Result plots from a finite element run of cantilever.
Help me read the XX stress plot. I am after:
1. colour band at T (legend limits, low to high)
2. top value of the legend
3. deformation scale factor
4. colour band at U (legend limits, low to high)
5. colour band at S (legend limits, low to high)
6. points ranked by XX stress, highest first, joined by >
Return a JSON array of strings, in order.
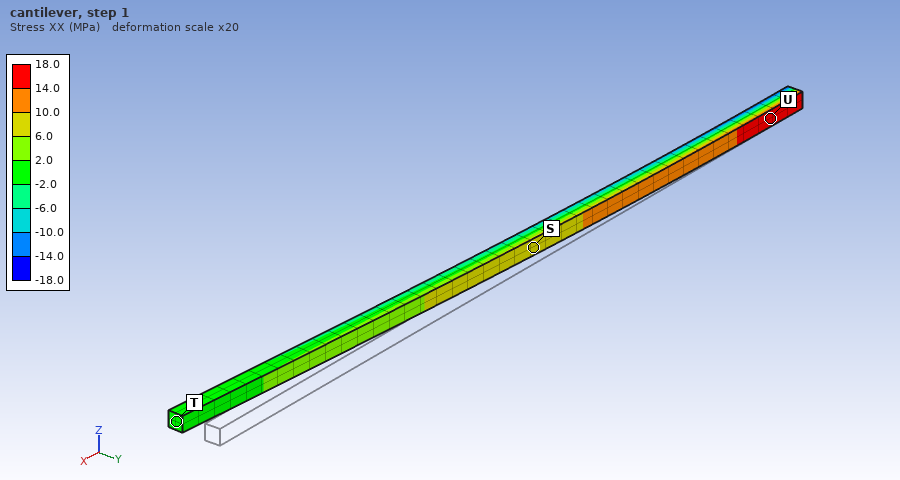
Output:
["-2.0 to 2.0 MPa", "18.0 MPa", "20", "14.0 to 18.0 MPa", "6.0 to 10.0 MPa", "U > S > T"]
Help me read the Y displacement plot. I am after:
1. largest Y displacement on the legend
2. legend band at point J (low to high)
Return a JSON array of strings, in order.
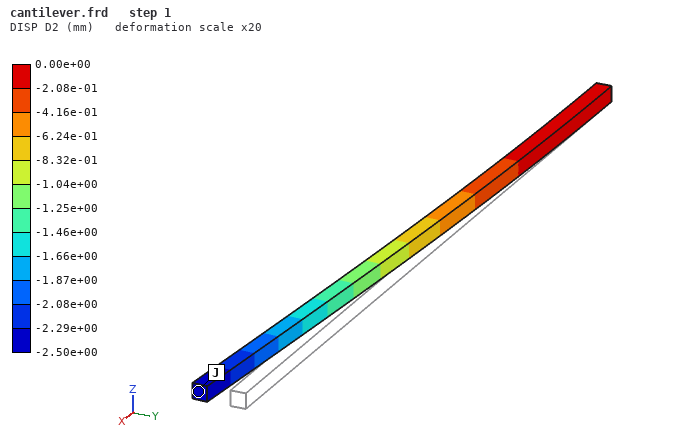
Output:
["0.00e+00 mm", "-2.50e+00 to -2.29e+00 mm"]
